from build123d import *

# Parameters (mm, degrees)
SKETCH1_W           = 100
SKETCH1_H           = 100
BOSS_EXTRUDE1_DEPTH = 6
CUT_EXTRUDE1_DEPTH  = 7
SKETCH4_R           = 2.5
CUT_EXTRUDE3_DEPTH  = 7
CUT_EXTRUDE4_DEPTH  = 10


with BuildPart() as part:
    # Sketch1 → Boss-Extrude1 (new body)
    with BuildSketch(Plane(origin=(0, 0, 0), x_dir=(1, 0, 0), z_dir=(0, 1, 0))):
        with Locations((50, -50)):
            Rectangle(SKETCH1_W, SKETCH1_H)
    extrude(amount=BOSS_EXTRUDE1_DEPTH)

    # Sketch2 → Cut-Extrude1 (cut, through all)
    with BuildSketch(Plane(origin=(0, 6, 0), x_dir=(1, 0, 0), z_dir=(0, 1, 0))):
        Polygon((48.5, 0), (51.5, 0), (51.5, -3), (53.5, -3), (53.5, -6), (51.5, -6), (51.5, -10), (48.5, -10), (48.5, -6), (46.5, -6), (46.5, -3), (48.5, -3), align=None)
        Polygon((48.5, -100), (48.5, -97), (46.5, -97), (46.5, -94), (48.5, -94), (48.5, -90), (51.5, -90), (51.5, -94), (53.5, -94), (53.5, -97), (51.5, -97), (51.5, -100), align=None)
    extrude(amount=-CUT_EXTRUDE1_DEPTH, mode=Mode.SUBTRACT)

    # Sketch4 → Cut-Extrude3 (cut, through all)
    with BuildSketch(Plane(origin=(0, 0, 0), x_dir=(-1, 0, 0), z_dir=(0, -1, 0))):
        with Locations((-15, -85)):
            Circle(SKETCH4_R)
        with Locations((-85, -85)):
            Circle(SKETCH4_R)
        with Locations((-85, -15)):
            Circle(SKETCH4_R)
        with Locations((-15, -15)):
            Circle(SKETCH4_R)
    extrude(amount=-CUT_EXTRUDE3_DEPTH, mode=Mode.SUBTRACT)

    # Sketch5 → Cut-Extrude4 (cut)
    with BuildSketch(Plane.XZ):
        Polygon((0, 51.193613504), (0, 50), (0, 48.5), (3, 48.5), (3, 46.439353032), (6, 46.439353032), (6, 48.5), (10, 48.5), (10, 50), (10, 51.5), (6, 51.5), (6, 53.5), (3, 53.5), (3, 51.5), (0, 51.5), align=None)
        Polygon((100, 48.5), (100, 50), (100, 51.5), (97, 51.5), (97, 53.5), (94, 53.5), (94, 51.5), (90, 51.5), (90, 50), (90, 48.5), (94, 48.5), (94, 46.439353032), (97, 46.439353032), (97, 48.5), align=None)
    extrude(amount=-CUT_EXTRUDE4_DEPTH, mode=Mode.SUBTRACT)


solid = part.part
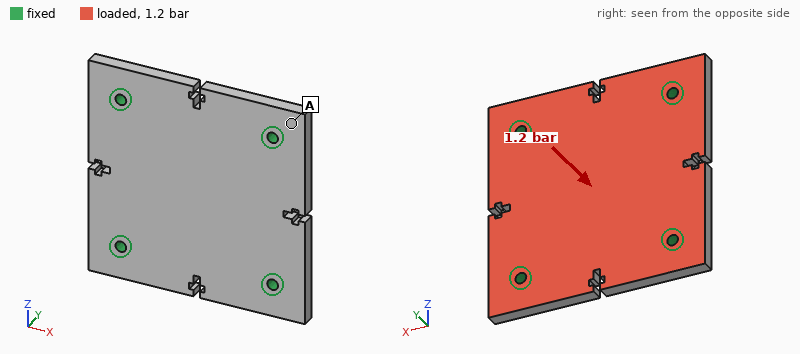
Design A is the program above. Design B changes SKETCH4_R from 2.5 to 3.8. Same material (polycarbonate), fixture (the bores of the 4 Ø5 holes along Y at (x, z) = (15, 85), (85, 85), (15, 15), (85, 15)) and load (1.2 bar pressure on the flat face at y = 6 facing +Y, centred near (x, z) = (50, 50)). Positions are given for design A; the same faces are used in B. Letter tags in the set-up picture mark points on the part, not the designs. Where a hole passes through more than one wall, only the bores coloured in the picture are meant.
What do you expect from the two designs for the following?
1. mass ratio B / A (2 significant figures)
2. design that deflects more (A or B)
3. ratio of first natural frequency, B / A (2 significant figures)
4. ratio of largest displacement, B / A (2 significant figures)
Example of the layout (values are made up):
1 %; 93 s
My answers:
0.99; A; 1.1; 0.83
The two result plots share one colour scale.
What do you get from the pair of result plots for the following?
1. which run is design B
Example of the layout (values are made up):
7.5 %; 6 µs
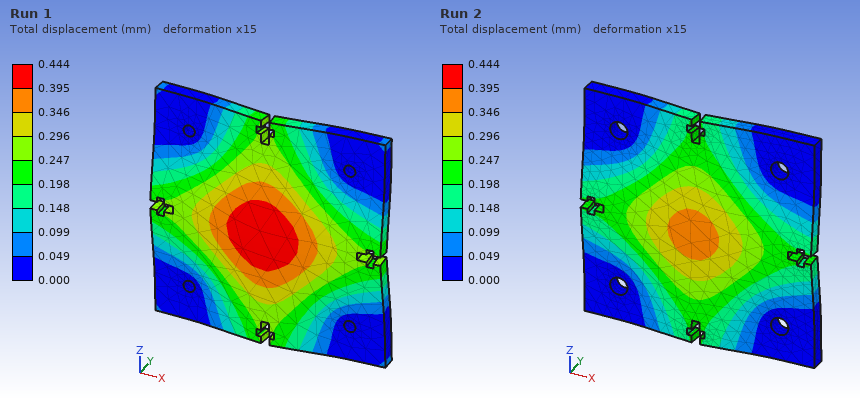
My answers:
Run 2
